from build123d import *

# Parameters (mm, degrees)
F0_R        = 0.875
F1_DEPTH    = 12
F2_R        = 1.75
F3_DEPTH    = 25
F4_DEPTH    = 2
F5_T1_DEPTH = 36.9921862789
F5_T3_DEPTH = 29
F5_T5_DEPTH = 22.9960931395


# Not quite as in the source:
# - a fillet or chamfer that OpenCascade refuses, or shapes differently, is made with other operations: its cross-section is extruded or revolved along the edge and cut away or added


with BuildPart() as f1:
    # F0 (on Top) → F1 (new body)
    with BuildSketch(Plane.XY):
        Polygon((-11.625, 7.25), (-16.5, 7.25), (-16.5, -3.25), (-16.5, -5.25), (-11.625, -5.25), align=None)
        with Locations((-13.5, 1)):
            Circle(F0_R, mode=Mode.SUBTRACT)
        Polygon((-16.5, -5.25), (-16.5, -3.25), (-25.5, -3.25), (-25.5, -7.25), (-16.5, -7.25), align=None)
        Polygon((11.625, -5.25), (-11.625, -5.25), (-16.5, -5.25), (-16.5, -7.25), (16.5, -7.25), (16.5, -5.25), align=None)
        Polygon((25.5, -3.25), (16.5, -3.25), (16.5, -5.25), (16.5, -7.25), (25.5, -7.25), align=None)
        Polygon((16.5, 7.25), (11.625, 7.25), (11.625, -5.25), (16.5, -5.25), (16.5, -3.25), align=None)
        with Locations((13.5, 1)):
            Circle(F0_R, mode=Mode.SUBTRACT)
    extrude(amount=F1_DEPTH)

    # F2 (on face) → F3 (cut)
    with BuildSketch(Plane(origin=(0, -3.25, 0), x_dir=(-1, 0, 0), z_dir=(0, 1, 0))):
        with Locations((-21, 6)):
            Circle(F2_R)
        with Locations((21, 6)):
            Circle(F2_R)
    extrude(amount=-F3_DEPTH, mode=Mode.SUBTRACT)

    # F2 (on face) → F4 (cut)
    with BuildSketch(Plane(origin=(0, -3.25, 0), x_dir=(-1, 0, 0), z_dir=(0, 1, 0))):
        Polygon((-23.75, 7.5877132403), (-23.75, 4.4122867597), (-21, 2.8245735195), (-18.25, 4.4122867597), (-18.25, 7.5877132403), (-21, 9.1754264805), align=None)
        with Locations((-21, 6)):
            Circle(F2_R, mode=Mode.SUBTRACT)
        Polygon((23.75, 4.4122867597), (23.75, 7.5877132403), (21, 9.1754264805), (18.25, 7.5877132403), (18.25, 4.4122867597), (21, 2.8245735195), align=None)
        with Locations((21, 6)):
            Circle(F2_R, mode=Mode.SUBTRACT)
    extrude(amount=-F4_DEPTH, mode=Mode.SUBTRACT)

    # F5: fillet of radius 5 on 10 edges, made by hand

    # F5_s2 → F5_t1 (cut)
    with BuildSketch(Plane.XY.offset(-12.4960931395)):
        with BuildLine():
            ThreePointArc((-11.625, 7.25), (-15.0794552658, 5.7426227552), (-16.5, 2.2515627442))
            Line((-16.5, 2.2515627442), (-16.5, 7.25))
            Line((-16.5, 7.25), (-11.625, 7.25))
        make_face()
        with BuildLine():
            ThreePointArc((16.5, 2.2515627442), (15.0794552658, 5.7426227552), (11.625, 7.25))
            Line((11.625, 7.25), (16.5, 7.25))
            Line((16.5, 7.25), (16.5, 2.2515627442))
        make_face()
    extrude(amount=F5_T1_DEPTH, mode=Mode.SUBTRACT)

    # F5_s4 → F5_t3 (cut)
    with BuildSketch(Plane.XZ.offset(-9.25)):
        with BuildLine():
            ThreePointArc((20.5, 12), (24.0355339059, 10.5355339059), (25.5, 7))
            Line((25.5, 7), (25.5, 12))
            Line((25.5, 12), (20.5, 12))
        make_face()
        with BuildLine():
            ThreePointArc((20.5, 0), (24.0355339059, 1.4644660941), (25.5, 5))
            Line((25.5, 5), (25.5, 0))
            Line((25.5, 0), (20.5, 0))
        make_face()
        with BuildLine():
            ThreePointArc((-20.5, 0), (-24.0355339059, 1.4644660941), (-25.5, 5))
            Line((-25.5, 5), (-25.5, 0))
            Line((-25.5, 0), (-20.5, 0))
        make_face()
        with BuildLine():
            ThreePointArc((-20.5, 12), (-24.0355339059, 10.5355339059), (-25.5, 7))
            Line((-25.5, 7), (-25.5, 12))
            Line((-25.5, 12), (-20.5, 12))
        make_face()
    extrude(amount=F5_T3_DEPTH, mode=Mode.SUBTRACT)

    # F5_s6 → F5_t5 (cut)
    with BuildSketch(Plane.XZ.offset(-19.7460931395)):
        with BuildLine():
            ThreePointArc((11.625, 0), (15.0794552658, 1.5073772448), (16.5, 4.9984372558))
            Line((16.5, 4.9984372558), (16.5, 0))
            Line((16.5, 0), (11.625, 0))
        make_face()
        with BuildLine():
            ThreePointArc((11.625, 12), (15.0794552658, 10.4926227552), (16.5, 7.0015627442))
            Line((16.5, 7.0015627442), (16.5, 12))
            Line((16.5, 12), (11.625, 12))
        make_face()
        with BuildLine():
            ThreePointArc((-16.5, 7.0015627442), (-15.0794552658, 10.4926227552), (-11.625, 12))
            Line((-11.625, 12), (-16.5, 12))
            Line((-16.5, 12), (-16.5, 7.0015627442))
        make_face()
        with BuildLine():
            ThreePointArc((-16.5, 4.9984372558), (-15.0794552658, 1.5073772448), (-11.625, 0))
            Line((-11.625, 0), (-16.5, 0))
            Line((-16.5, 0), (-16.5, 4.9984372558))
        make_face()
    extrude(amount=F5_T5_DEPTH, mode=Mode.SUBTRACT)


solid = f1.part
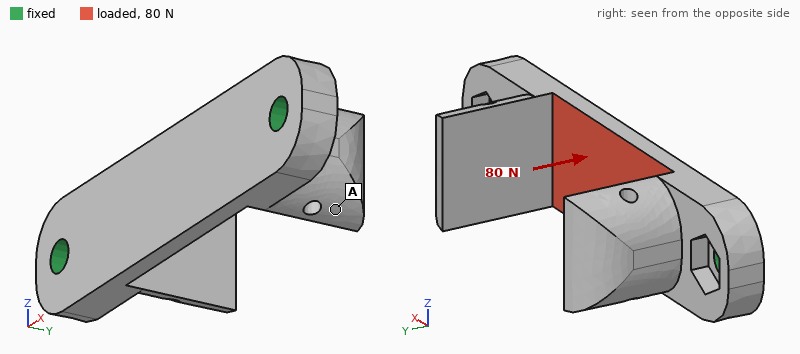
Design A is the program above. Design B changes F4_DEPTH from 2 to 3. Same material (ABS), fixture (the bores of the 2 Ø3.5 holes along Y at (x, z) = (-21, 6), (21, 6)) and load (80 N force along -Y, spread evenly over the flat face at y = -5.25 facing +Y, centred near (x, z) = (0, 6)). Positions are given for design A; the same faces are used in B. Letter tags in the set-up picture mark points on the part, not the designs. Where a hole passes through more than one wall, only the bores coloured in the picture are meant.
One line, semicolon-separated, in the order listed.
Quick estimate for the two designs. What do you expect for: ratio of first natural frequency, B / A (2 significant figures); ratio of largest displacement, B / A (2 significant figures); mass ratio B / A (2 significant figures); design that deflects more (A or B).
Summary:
0.73; 1.6; 0.99; B
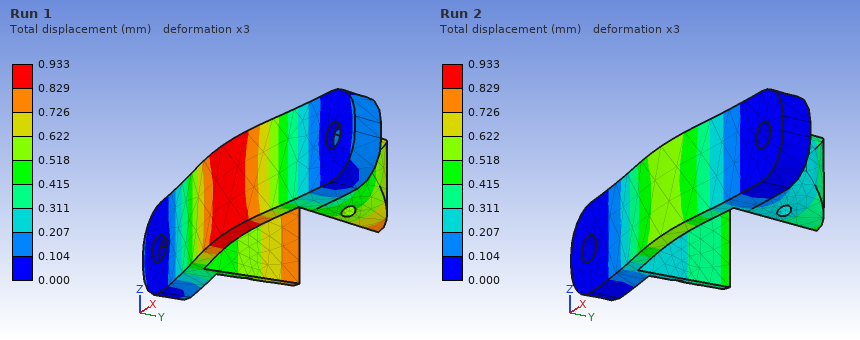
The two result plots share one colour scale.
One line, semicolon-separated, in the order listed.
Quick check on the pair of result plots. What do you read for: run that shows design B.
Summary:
Run 1
